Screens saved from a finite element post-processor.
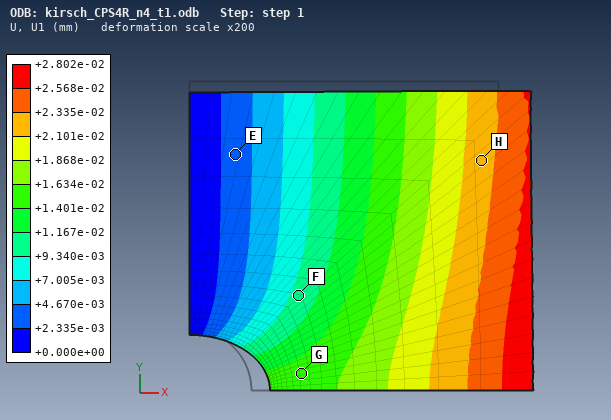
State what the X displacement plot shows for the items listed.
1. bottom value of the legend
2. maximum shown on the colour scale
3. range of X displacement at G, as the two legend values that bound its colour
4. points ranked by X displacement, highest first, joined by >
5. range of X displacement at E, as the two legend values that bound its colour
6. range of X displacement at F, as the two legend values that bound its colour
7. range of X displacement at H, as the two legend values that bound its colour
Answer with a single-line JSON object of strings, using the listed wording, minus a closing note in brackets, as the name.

{"bottom value of the legend": "+0.000e+00 mm", "maximum shown on the colour scale": "+2.802e-02 mm", "range of X displacement at G, as the two legend values that bound its colour": "+1.401e-02 to +1.634e-02 mm", "points ranked by X displacement, highest first, joined by >": "H > G > F > E", "range of X displacement at E, as the two legend values that bound its colour": "+2.335e-03 to +4.670e-03 mm", "range of X displacement at F, as the two legend values that bound its colour": "+9.340e-03 to +1.167e-02 mm", "range of X displacement at H, as the two legend values that bound its colour": "+2.101e-02 to +2.335e-02 mm"}
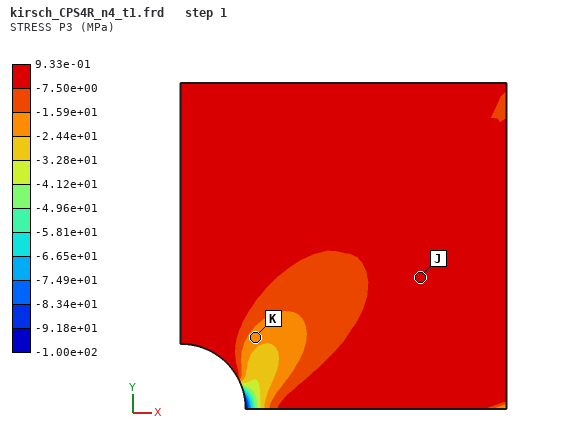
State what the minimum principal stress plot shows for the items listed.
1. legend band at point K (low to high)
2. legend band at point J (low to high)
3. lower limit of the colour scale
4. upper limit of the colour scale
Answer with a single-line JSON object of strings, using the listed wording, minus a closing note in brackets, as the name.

{"legend band at point K": "-2.44e+01 to -1.59e+01 MPa", "legend band at point J": "-7.50e+00 to 9.33e-01 MPa", "lower limit of the colour scale": "-1.00e+02 MPa", "upper limit of the colour scale": "9.33e-01 MPa"}
